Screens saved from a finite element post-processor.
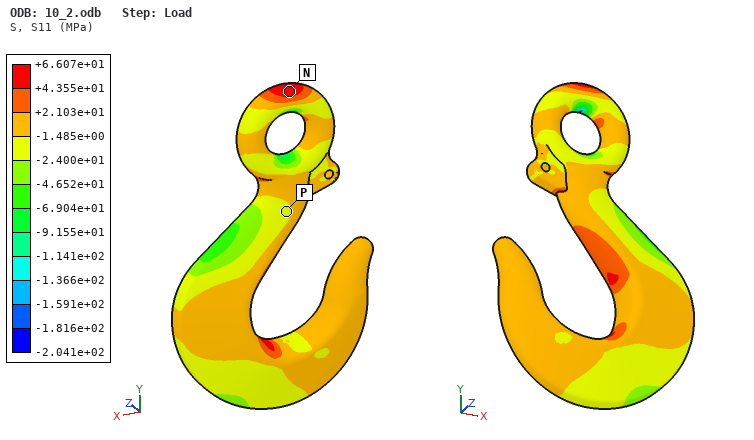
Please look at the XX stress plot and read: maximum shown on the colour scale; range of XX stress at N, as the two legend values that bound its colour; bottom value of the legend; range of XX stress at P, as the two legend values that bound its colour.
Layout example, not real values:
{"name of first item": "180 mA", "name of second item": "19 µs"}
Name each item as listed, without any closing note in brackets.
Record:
{"maximum shown on the colour scale": "+6.607e+01 MPa", "range of XX stress at N, as the two legend values that bound its colour": "+4.355e+01 to +6.607e+01 MPa", "bottom value of the legend": "-2.041e+02 MPa", "range of XX stress at P, as the two legend values that bound its colour": "-2.400e+01 to -1.485e+00 MPa"}
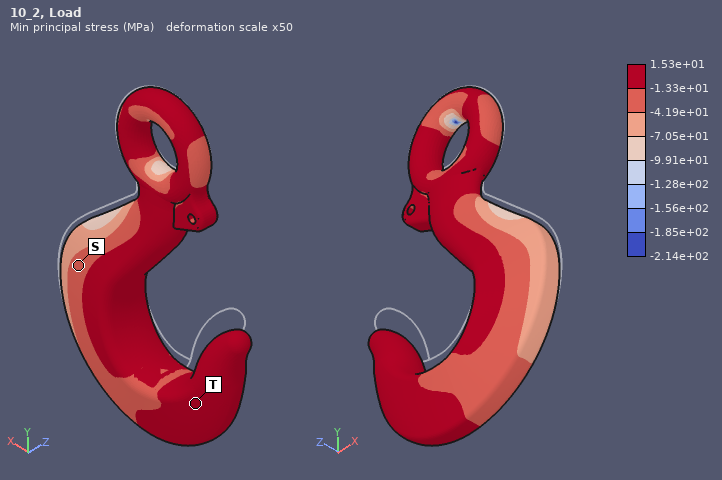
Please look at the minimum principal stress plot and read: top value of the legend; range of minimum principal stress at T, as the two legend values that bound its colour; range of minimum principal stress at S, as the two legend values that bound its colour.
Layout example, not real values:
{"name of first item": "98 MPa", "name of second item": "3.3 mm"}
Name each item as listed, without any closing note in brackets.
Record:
{"top value of the legend": "1.53e+01 MPa", "range of minimum principal stress at T, as the two legend values that bound its colour": "-1.33e+01 to 1.53e+01 MPa", "range of minimum principal stress at S, as the two legend values that bound its colour": "-4.19e+01 to -1.33e+01 MPa"}
